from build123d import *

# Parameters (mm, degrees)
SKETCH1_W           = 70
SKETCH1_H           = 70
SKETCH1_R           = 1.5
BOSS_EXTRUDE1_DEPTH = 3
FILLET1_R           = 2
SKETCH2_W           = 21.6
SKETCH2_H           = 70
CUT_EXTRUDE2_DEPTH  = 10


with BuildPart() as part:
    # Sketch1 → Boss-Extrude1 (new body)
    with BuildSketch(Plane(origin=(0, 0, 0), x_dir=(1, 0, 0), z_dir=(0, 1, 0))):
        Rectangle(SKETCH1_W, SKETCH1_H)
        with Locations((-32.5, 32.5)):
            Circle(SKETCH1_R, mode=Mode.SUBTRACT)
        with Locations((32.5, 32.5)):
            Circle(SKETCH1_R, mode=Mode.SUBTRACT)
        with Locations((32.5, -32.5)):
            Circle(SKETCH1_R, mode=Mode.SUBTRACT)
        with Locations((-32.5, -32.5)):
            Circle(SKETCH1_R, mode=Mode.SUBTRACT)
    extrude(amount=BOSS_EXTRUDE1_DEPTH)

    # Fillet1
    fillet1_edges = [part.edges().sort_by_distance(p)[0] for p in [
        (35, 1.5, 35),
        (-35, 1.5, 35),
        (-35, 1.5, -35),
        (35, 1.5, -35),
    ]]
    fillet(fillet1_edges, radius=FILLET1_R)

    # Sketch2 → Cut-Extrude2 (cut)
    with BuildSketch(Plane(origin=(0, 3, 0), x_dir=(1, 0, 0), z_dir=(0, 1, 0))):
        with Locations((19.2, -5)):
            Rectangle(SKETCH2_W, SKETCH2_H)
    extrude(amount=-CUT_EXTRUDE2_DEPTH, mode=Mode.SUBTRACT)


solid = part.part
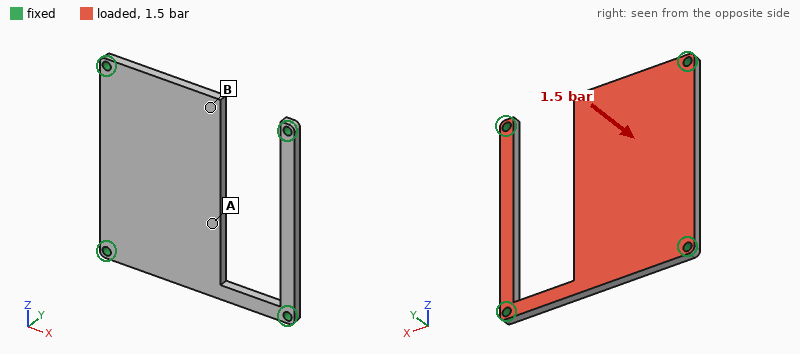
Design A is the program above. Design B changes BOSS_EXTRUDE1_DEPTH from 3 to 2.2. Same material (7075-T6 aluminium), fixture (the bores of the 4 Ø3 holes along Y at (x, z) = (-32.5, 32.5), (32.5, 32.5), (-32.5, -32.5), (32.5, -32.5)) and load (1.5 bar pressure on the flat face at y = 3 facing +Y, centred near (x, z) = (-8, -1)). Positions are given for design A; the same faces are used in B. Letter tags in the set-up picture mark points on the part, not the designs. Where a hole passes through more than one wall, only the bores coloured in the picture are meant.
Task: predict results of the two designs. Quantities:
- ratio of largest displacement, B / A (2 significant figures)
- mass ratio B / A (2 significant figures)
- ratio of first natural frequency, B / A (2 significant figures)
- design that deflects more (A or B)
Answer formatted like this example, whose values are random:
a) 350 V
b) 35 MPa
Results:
a) 2.4
b) 0.73
c) 0.75
d) B
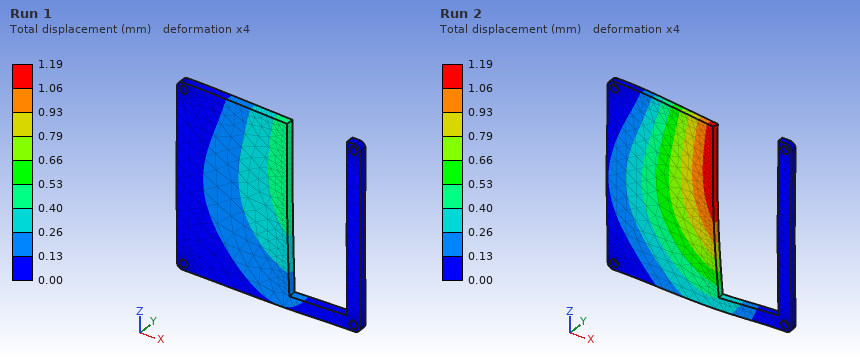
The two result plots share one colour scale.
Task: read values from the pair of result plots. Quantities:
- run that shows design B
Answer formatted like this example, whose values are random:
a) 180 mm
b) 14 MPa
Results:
a) Run 2
